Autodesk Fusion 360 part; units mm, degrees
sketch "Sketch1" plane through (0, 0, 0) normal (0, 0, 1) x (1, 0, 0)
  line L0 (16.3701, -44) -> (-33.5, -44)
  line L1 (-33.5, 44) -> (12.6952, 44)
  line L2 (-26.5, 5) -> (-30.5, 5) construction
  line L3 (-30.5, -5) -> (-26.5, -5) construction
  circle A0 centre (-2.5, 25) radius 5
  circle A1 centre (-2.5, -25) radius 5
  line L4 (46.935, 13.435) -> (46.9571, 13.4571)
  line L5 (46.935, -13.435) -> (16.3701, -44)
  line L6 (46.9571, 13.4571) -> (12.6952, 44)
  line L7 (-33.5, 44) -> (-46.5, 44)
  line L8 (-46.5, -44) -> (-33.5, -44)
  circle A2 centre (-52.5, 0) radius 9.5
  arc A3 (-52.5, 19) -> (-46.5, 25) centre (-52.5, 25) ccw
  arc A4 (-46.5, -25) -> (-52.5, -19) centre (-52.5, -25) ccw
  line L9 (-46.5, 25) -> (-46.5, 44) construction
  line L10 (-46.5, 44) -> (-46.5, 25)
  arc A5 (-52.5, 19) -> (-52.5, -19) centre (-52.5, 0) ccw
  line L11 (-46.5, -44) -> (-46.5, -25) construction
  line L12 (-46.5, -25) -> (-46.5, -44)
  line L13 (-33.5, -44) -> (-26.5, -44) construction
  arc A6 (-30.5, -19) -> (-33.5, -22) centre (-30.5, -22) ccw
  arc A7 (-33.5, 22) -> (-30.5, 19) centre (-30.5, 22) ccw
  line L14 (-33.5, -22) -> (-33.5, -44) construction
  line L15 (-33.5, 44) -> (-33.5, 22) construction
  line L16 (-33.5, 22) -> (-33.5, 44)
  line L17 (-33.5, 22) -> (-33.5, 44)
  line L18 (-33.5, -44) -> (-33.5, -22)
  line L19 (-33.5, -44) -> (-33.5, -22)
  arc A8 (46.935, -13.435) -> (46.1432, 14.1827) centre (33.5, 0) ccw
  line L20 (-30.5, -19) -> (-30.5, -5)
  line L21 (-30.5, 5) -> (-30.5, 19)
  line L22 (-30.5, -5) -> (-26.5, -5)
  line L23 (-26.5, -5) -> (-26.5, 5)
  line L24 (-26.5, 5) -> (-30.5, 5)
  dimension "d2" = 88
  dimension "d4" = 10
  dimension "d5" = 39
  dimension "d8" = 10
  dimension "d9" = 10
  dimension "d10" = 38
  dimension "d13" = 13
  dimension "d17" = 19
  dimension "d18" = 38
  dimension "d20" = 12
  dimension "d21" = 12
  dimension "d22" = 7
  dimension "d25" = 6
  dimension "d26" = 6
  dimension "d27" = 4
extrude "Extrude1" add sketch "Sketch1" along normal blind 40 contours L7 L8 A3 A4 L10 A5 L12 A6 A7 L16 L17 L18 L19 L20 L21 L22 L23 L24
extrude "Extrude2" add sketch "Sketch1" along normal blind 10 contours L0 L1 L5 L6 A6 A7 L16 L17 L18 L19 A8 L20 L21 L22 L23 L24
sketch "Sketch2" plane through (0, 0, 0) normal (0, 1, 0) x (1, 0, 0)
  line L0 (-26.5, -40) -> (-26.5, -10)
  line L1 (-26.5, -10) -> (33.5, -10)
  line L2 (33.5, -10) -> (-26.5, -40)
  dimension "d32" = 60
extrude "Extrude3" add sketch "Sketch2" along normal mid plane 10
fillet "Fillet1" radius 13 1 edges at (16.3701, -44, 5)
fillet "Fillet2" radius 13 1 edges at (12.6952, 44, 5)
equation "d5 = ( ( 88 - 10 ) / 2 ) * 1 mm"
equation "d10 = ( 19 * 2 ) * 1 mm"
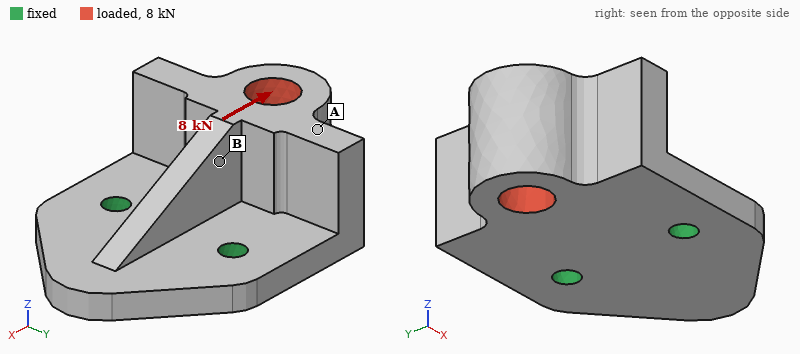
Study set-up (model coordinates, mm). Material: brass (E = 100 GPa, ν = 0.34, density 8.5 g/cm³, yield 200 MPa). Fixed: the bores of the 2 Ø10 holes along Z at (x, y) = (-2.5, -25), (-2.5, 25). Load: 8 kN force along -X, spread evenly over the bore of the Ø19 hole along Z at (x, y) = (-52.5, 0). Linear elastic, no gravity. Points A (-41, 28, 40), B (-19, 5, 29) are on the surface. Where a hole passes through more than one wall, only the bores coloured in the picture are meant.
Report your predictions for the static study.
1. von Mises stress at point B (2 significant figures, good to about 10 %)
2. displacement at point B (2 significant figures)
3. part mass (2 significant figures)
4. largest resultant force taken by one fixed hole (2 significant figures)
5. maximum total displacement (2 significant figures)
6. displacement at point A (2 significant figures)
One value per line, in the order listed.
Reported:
23 MPa
0.043 mm
1.2 kg
4.0 kN
0.12 mm
0.080 mm
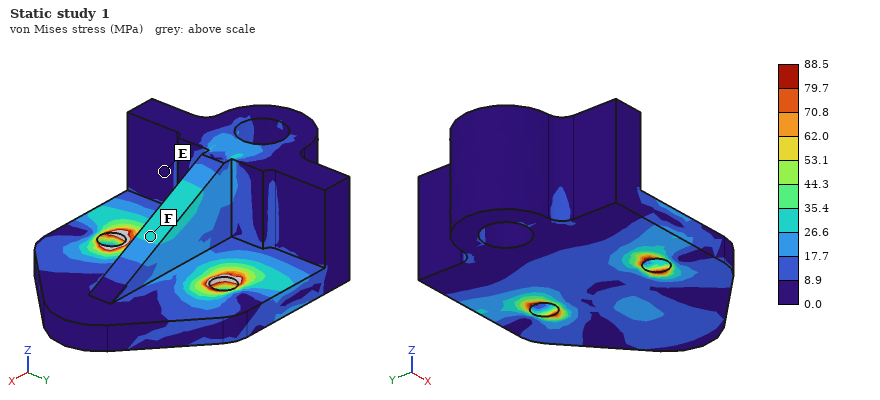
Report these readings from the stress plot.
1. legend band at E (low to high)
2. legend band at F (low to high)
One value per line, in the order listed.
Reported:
0.0 to 8.9 MPa
26.6 to 35.4 MPa
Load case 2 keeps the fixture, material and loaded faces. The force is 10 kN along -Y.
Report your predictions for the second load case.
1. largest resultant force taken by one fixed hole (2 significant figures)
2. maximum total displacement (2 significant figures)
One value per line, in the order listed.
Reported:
11 kN
68 µm
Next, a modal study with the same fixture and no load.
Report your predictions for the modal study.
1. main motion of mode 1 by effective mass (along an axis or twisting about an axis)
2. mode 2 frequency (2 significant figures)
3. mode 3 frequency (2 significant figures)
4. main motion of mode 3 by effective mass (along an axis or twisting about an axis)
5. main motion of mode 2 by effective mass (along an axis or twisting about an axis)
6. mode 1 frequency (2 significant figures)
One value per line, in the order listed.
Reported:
along Z
2400 Hz
3500 Hz
along Z
along Y
1200 Hz
